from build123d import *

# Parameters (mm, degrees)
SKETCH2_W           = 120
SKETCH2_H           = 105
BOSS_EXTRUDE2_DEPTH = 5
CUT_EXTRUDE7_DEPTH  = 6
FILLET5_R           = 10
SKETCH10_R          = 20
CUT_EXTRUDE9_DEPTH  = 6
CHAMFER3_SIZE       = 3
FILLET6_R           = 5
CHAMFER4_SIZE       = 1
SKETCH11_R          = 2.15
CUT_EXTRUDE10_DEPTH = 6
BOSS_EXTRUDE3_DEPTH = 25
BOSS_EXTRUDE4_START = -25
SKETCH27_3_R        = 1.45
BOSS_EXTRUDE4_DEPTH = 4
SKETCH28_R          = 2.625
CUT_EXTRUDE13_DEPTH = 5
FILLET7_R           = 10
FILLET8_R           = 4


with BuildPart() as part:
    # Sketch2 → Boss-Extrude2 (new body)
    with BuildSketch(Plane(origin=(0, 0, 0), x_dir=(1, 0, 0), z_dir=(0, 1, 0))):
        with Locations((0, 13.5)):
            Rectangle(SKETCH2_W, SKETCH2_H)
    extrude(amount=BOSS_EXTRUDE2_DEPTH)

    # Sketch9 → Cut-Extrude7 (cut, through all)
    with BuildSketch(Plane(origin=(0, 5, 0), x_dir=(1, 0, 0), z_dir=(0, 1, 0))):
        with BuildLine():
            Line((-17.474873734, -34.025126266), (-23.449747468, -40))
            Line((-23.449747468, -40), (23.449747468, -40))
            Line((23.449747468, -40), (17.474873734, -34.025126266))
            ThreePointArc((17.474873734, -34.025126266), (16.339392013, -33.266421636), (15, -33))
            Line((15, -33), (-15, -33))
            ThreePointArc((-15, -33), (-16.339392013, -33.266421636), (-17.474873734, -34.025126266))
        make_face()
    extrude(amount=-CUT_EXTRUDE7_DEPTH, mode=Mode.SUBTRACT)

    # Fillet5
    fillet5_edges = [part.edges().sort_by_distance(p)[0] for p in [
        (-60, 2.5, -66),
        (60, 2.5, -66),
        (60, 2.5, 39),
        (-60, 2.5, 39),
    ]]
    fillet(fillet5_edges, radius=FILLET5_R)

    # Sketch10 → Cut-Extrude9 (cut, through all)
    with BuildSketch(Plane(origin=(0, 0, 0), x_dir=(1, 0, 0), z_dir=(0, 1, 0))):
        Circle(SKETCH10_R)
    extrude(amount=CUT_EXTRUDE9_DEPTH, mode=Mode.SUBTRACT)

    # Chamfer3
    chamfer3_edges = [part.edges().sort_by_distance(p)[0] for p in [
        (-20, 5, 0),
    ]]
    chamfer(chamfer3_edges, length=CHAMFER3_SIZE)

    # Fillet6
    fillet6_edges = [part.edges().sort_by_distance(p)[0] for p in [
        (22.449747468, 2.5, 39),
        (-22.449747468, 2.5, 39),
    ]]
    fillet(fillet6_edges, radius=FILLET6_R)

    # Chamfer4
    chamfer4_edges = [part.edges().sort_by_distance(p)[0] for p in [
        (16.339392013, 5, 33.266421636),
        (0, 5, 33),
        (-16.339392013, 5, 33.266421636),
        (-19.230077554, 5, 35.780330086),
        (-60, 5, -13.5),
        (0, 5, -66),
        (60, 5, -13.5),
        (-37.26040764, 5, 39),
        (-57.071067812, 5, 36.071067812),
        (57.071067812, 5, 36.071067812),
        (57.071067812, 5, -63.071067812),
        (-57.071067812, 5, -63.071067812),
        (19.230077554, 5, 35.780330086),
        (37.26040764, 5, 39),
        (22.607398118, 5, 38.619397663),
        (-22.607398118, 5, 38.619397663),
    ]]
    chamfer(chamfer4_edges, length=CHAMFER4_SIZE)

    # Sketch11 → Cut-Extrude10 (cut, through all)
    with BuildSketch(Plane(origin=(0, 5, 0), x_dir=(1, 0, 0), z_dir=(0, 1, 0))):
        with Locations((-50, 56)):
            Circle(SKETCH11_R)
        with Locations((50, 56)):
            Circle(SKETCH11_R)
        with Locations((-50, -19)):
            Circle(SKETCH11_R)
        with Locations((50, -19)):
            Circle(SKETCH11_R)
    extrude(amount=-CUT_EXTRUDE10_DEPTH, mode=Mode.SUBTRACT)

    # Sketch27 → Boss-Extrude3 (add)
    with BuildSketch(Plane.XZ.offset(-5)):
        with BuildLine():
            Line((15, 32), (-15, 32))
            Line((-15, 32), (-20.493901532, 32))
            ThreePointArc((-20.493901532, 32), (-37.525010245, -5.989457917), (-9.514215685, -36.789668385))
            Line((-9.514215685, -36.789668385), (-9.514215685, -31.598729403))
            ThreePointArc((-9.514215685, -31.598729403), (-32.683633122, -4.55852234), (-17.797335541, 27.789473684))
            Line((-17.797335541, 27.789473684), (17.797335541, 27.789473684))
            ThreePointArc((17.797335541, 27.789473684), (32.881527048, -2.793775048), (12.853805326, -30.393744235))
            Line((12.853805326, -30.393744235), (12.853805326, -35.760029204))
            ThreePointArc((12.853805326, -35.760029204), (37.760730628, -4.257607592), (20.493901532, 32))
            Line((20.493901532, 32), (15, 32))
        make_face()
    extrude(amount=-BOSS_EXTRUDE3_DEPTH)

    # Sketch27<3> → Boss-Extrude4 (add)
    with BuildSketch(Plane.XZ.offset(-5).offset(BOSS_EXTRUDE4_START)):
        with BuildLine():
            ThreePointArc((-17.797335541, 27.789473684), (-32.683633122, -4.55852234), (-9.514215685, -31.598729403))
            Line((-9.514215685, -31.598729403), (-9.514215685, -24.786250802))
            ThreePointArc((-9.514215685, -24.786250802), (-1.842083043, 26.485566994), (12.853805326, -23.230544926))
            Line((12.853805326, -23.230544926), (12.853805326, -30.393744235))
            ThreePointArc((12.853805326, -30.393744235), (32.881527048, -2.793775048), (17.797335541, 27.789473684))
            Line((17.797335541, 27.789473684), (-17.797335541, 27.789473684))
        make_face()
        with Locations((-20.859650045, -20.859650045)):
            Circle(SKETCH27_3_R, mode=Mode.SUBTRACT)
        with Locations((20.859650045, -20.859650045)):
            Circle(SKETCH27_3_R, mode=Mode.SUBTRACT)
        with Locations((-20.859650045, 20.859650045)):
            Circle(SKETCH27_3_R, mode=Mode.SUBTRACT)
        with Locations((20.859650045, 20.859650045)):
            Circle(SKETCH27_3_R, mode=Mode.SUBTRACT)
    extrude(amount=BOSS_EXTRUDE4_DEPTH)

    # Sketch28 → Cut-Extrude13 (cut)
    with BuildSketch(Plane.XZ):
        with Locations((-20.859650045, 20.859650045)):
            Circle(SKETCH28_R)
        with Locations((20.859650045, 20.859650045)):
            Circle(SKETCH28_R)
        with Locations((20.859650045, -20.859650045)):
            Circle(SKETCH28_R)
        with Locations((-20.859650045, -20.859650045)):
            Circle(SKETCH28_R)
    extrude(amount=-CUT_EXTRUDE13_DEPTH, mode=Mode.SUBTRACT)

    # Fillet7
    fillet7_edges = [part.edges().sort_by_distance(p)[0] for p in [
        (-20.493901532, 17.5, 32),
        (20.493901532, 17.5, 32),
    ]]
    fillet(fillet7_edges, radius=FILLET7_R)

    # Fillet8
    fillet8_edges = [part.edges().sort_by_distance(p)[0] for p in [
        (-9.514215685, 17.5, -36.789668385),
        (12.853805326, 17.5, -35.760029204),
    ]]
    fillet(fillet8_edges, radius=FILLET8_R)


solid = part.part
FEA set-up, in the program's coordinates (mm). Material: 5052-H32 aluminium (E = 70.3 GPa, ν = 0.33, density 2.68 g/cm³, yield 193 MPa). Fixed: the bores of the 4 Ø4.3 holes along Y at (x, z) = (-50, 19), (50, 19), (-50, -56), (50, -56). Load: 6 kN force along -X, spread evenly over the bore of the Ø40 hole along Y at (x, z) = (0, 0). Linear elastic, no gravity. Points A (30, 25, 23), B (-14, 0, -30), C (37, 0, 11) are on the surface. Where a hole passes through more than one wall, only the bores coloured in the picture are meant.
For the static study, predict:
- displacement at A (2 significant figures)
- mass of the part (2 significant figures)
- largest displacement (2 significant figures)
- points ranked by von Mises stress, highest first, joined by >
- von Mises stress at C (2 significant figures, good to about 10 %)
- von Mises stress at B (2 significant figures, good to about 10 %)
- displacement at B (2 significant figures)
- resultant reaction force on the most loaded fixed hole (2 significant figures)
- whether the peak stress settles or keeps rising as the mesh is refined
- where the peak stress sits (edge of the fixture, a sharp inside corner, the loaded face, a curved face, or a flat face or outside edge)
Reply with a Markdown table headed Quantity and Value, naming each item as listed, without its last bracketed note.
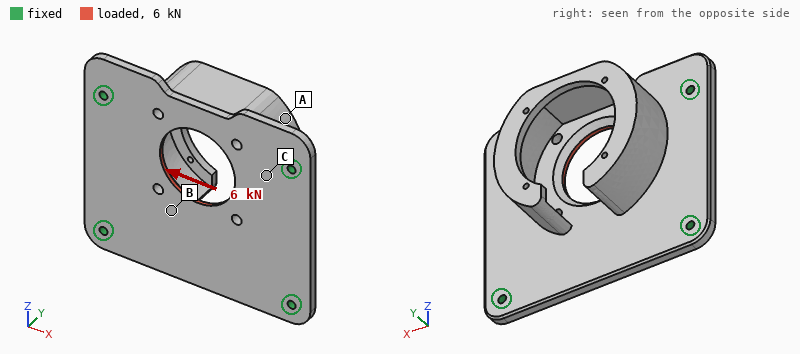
| Quantity | Value |
|---|---|
| displacement at A | 4.8 µm |
| mass of the part | 220 g |
| largest displacement | 13 µm |
| points ranked by von Mises stress, highest first, joined by > | C > B > A |
| von Mises stress at C | 18 MPa |
| von Mises stress at B | 8.1 MPa |
| displacement at B | 6.9 µm |
| resultant reaction force on the most loaded fixed hole | 2.0 kN |
| whether the peak stress settles or keeps rising as the mesh is refined | keeps rising |
| where the peak stress sits | edge of the fixture |
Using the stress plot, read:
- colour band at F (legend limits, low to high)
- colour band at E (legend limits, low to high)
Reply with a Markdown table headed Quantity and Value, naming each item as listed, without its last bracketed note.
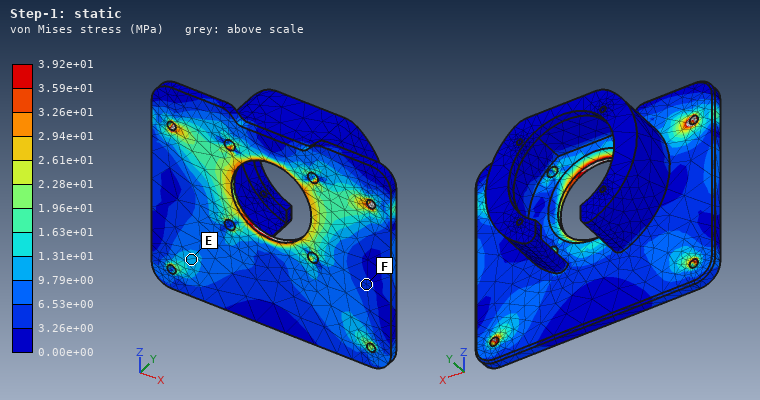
| Quantity | Value |
|---|---|
| colour band at F | 3.26e+00 to 6.53e+00 MPa |
| colour band at E | 9.79e+00 to 1.31e+01 MPa |
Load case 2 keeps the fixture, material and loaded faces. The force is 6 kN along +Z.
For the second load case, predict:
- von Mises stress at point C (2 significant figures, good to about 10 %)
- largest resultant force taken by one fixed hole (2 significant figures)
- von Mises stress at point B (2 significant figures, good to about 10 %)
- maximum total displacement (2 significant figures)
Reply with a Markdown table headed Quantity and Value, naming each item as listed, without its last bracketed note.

| Quantity | Value |
|---|---|
| von Mises stress at point C | 14 MPa |
| largest resultant force taken by one fixed hole | 1.6 kN |
| von Mises stress at point B | 14 MPa |
| maximum total displacement | 34 µm |
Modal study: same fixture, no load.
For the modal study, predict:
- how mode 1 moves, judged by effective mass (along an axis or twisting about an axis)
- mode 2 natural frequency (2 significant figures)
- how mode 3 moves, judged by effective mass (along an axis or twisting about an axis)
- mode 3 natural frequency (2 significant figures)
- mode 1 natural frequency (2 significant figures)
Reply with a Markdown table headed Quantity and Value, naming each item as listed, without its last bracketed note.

| Quantity | Value |
|---|---|
| how mode 1 moves, judged by effective mass | along Y |
| mode 2 natural frequency | 3000 Hz |
| how mode 3 moves, judged by effective mass | twisting about Z |
| mode 3 natural frequency | 4000 Hz |
| mode 1 natural frequency | 2000 Hz |
